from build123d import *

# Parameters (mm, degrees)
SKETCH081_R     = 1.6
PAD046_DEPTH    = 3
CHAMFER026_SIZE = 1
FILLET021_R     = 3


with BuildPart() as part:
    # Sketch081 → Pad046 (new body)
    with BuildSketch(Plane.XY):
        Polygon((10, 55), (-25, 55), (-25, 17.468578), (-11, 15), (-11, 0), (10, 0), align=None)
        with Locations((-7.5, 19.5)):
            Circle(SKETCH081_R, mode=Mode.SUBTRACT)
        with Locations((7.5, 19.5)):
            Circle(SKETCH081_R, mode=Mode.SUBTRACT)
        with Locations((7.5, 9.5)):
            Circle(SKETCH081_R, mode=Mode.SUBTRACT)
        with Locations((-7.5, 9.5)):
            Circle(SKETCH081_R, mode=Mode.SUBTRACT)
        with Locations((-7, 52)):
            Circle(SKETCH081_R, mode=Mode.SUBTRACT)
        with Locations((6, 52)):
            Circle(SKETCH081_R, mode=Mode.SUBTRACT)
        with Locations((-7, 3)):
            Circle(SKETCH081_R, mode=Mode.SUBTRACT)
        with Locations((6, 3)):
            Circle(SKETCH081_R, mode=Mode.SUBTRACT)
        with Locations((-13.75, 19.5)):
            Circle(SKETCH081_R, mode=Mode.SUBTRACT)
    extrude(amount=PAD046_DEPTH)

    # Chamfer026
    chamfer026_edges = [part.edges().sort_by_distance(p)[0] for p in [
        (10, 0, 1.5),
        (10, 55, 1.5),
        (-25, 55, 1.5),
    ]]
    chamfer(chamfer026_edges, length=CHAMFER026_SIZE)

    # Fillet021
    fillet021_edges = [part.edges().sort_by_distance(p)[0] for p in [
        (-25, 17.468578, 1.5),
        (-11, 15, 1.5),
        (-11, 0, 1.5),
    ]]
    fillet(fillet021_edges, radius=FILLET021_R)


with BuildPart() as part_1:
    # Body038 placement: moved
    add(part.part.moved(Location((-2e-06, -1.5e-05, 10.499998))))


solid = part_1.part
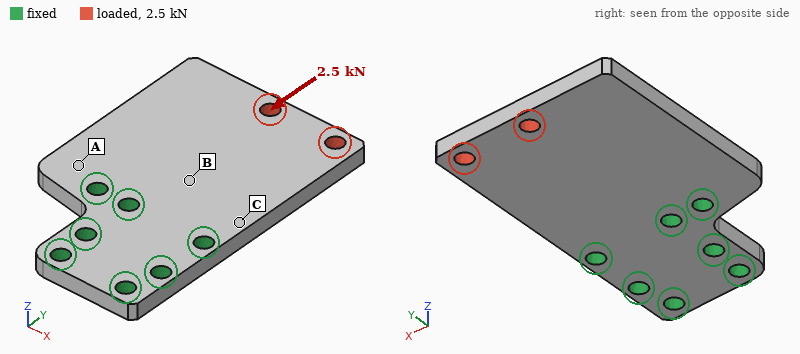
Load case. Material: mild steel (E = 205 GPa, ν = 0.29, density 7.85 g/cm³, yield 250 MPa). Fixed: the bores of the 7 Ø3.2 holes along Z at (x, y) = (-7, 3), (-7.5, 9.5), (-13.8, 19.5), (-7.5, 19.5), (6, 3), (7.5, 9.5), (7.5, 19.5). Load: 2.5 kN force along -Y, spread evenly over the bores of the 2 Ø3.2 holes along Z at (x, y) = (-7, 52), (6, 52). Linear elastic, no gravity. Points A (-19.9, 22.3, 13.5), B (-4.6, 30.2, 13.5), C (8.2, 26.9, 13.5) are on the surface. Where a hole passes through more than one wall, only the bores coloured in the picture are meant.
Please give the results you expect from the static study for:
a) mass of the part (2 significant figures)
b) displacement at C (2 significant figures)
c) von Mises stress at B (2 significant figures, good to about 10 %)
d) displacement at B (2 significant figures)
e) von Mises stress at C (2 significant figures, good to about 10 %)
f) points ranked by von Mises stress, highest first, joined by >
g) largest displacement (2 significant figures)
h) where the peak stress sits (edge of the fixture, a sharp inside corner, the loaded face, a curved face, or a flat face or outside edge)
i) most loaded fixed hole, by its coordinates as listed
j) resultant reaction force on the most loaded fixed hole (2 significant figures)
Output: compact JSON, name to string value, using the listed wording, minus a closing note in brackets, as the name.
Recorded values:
{"mass of the part": "38 g", "displacement at C": "1.9 µm", "von Mises stress at B": "28 MPa", "displacement at B": "1.6 µm", "von Mises stress at C": "53 MPa", "points ranked by von Mises stress, highest first, joined by >": "C > B > A", "largest displacement": "10 µm", "where the peak stress sits": "the loaded face", "most loaded fixed hole, by its coordinates as listed": "(7.5, 19.5)", "resultant reaction force on the most loaded fixed hole": "1.2 kN"}
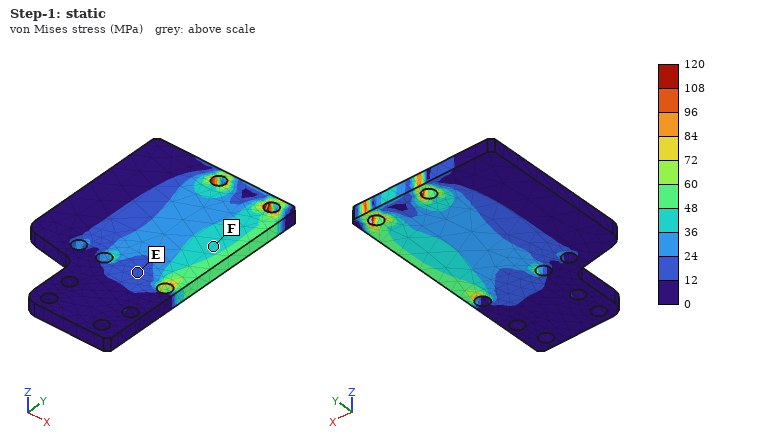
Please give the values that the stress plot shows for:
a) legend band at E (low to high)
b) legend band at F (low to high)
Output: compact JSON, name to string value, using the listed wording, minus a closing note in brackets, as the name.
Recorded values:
{"legend band at E": "12 to 24 MPa", "legend band at F": "36 to 48 MPa"}
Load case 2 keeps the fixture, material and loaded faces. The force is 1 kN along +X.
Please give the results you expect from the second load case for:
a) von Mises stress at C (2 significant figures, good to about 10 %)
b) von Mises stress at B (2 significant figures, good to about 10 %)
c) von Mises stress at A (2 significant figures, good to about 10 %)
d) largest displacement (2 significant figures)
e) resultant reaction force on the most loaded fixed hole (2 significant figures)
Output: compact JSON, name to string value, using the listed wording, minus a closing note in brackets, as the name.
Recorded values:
{"von Mises stress at C": "55 MPa", "von Mises stress at B": "31 MPa", "von Mises stress at A": "22 MPa", "largest displacement": "17 µm", "resultant reaction force on the most loaded fixed hole": "1.4 kN"}
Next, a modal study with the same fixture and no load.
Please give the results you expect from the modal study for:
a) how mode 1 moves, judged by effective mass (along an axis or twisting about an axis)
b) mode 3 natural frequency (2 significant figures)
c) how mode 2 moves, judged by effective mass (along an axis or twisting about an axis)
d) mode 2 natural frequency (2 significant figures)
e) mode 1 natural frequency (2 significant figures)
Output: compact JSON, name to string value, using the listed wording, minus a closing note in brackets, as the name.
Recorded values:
{"how mode 1 moves, judged by effective mass": "along Z", "mode 3 natural frequency": "11 kHz", "how mode 2 moves, judged by effective mass": "twisting about Y", "mode 2 natural frequency": "4700 Hz", "mode 1 natural frequency": "2000 Hz"}
